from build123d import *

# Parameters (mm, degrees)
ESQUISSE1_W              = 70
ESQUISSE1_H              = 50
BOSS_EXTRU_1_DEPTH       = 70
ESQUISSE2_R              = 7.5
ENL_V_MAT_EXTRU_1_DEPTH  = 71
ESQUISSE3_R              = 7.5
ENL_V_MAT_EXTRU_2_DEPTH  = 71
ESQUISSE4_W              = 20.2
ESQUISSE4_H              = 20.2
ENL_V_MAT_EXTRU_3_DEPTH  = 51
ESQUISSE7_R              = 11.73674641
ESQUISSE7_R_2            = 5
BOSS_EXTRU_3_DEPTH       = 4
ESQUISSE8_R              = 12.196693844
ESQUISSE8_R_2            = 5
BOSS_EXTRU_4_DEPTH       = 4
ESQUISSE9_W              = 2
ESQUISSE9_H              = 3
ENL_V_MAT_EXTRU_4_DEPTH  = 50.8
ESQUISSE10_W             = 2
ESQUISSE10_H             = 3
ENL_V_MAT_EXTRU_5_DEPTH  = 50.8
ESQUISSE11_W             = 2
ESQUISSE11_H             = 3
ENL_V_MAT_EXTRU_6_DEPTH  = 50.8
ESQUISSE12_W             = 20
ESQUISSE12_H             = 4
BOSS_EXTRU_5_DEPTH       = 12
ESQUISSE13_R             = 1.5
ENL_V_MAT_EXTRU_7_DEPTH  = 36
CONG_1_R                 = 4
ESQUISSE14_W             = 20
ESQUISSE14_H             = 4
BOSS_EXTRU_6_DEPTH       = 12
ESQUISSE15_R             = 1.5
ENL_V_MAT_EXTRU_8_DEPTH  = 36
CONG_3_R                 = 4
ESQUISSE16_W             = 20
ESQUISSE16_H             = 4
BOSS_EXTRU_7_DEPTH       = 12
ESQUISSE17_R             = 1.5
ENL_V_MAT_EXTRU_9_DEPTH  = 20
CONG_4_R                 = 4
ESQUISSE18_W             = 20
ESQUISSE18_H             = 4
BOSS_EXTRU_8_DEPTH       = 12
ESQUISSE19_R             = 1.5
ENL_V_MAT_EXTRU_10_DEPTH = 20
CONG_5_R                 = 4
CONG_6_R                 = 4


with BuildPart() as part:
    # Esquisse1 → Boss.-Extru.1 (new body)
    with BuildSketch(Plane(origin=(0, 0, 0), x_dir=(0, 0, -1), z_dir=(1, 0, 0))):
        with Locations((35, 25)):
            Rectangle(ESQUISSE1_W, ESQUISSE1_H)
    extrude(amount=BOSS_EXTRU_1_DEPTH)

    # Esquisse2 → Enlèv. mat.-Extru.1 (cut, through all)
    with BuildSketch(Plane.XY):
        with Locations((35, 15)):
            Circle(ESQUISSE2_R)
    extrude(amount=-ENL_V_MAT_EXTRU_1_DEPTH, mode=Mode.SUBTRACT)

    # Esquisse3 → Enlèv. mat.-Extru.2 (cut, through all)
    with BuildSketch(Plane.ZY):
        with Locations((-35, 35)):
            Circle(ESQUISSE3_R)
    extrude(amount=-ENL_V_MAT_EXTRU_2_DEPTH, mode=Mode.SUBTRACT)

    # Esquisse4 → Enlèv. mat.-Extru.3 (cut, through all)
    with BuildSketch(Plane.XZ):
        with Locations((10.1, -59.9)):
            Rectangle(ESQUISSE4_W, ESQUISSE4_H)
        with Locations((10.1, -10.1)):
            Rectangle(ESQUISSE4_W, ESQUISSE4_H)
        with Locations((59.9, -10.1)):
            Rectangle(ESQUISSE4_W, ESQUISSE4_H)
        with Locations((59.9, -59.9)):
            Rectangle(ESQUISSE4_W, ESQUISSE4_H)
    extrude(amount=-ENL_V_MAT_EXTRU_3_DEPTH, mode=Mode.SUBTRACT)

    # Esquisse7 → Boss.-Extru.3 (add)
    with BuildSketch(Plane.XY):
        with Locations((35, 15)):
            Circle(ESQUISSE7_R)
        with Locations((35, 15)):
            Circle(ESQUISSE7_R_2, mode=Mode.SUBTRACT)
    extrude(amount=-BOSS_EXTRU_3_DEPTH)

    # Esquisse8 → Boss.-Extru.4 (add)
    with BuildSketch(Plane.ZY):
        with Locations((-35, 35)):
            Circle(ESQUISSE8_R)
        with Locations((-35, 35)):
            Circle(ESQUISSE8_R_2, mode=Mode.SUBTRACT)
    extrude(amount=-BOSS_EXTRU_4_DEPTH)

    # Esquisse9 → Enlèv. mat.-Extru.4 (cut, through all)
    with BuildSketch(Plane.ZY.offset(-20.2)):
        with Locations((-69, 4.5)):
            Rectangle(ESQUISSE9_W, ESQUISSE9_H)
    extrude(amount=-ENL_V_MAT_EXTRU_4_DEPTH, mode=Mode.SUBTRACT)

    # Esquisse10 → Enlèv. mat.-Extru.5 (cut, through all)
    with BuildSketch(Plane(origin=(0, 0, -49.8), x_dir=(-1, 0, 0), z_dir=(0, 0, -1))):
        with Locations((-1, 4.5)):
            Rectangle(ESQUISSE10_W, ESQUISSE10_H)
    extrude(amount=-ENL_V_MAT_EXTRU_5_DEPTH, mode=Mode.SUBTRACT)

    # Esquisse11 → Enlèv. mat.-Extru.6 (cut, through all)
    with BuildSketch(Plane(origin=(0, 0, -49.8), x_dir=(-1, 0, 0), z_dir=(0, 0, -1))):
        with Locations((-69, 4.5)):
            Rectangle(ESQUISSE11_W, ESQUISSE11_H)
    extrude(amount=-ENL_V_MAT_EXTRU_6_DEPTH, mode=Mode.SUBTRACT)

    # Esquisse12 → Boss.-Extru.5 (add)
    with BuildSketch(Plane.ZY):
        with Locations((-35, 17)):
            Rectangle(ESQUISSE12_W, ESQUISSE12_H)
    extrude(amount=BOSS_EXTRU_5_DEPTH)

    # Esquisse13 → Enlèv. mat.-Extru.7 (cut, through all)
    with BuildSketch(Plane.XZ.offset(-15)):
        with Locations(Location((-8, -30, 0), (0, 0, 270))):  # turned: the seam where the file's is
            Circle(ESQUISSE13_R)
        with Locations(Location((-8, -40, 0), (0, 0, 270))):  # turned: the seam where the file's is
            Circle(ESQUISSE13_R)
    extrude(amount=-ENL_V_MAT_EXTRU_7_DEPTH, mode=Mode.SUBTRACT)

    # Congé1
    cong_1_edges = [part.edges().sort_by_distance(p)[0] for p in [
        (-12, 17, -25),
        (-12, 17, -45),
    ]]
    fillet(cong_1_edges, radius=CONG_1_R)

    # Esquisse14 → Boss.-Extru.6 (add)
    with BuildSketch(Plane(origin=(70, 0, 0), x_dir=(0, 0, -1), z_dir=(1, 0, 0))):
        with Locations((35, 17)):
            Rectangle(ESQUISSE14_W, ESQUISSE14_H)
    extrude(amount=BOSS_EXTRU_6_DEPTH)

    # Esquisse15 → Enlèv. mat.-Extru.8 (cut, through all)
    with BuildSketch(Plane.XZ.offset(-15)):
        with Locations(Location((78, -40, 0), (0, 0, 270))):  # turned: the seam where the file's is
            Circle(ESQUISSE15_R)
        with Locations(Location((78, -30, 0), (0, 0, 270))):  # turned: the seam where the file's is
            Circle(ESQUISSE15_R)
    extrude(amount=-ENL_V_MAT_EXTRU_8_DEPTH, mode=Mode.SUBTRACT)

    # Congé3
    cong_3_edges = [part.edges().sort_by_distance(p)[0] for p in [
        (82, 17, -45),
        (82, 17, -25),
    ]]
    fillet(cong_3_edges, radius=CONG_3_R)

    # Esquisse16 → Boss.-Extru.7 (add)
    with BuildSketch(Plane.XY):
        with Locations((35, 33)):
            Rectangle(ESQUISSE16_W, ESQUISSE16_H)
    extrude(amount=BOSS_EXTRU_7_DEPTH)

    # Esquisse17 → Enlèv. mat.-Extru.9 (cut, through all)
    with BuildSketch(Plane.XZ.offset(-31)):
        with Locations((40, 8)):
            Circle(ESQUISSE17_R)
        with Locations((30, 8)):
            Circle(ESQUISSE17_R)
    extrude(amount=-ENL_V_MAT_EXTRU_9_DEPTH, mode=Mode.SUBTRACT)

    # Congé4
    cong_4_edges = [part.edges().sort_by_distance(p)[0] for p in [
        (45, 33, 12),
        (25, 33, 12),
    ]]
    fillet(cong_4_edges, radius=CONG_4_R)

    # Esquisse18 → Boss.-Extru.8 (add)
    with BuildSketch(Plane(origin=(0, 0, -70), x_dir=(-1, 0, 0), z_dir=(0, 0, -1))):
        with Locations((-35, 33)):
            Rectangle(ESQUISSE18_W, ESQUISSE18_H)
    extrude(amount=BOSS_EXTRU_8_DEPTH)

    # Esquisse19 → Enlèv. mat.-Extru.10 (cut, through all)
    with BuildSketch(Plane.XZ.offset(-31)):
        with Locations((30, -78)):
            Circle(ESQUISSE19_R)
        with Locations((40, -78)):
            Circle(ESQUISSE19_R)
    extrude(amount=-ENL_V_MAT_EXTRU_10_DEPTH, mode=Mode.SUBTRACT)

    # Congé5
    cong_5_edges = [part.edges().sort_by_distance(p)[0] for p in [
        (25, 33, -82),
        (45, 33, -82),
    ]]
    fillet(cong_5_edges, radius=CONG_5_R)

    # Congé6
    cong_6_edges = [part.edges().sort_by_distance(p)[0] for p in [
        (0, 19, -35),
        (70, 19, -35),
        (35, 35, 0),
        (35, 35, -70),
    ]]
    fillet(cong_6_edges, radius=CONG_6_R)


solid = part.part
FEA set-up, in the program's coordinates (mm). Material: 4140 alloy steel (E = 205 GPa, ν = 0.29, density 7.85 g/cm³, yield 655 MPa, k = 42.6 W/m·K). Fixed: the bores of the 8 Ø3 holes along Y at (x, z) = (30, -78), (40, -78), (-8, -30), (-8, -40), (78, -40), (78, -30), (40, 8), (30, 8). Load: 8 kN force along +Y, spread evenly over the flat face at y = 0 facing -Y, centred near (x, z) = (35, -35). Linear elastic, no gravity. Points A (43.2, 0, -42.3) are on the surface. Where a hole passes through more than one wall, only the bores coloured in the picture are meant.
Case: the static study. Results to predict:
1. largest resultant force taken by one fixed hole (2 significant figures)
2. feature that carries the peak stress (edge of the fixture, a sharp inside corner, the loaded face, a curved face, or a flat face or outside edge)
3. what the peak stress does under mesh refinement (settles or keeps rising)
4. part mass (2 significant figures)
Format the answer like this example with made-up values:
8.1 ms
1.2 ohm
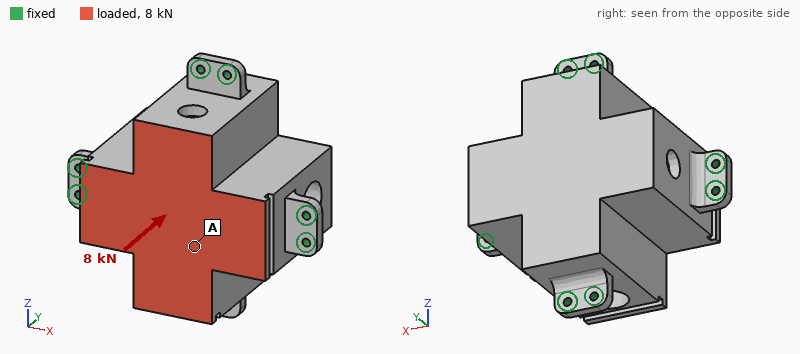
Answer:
1.0 kN
edge of the fixture
keeps rising
1.1 kg
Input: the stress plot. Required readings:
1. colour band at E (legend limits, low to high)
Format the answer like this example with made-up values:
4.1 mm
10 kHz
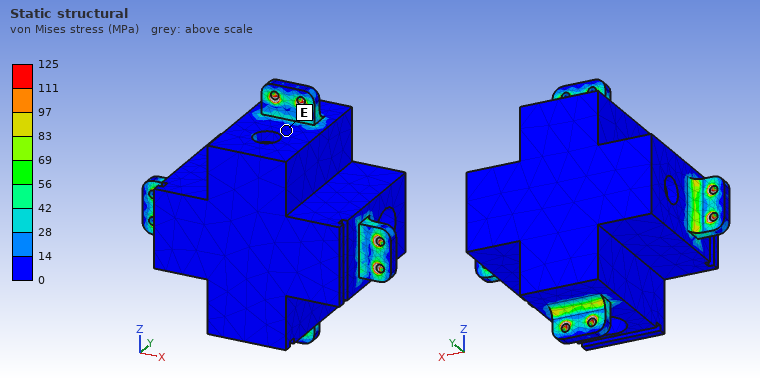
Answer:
0 to 14 MPa
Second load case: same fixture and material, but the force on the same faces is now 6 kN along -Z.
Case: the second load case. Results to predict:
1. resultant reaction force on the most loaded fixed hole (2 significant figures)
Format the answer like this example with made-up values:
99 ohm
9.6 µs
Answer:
1.1 kN
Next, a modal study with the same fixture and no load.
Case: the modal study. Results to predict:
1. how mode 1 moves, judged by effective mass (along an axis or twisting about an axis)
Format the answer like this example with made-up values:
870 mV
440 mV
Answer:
along Y
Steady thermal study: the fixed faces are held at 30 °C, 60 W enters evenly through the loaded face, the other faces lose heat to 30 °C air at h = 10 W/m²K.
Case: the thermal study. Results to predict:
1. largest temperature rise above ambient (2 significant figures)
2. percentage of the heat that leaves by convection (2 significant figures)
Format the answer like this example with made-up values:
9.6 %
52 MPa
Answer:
52 K
15 %
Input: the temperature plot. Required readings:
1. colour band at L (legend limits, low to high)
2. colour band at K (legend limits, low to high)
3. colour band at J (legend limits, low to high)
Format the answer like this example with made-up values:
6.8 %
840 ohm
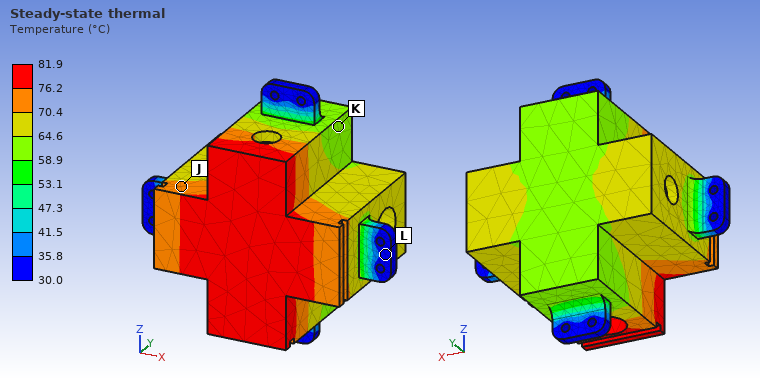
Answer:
30.0 to 35.8 °C
58.9 to 64.6 °C
70.4 to 76.2 °C
